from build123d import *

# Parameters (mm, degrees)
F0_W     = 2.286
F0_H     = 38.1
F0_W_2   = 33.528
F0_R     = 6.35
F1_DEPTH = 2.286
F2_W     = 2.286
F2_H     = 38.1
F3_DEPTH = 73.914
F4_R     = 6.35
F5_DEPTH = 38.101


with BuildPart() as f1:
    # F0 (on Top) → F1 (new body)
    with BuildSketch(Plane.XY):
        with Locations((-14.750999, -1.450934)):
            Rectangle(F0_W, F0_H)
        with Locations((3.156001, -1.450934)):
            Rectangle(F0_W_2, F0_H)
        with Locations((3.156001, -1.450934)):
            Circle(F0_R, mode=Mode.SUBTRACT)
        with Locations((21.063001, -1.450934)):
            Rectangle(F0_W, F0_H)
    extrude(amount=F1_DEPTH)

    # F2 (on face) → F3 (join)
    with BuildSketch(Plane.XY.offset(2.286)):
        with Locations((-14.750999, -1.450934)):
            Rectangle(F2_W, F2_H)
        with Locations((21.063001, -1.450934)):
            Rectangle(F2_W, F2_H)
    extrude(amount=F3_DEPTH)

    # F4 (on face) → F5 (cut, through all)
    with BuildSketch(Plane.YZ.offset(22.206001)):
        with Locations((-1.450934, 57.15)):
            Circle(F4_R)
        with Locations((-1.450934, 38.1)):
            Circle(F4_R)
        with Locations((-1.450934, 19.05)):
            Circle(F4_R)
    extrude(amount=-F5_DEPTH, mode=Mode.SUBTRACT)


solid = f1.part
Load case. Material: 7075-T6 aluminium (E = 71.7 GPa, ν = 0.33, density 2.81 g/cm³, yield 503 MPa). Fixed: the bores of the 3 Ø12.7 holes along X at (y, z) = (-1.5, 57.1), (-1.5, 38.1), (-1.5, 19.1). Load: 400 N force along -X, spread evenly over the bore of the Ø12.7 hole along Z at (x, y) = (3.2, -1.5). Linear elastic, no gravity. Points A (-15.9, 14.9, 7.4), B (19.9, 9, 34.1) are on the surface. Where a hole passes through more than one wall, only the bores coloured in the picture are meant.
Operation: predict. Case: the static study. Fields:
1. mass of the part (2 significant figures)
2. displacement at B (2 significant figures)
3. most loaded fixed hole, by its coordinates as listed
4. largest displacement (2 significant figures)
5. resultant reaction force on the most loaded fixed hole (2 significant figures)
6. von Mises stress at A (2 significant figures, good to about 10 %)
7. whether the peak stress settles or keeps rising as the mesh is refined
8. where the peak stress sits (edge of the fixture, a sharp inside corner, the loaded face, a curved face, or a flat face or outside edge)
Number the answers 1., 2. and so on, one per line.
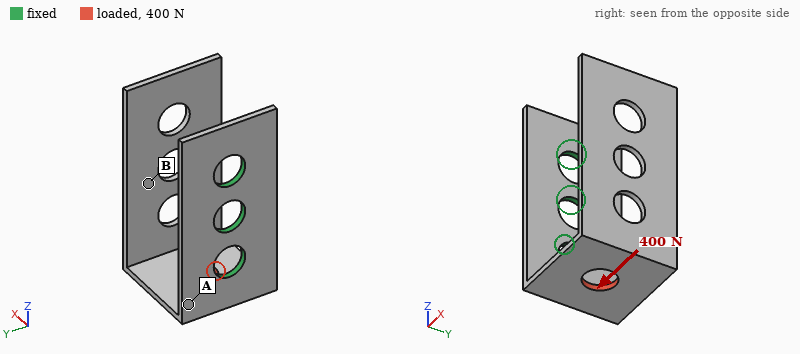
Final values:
1. 40 g
2. 0.54 mm
3. (-1.5, 19.1)
4. 0.98 mm
5. 420 N
6. 53 MPa
7. keeps rising
8. edge of the fixture
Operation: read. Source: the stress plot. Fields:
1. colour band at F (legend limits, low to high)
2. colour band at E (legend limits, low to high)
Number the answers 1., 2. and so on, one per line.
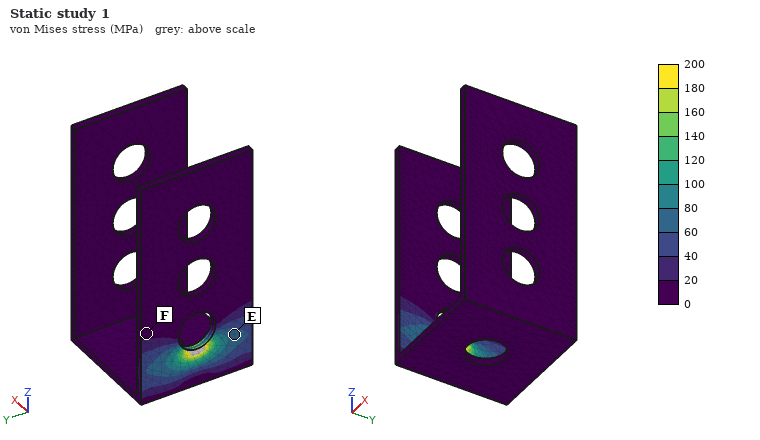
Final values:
1. 0 to 20 MPa
2. 60 to 80 MPa
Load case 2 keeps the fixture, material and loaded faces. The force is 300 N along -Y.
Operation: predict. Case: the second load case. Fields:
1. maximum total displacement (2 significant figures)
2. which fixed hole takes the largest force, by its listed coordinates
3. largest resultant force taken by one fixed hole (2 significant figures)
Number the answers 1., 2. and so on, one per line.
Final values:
1. 0.79 mm
2. (-1.5, 19.1)
3. 380 N
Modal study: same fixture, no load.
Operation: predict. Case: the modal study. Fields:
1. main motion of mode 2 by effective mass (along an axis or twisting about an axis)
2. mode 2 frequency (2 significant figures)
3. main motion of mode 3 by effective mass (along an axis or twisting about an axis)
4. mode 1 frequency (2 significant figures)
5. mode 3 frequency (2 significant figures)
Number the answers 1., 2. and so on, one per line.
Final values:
1. along Y
2. 280 Hz
3. along Z
4. 170 Hz
5. 530 Hz
